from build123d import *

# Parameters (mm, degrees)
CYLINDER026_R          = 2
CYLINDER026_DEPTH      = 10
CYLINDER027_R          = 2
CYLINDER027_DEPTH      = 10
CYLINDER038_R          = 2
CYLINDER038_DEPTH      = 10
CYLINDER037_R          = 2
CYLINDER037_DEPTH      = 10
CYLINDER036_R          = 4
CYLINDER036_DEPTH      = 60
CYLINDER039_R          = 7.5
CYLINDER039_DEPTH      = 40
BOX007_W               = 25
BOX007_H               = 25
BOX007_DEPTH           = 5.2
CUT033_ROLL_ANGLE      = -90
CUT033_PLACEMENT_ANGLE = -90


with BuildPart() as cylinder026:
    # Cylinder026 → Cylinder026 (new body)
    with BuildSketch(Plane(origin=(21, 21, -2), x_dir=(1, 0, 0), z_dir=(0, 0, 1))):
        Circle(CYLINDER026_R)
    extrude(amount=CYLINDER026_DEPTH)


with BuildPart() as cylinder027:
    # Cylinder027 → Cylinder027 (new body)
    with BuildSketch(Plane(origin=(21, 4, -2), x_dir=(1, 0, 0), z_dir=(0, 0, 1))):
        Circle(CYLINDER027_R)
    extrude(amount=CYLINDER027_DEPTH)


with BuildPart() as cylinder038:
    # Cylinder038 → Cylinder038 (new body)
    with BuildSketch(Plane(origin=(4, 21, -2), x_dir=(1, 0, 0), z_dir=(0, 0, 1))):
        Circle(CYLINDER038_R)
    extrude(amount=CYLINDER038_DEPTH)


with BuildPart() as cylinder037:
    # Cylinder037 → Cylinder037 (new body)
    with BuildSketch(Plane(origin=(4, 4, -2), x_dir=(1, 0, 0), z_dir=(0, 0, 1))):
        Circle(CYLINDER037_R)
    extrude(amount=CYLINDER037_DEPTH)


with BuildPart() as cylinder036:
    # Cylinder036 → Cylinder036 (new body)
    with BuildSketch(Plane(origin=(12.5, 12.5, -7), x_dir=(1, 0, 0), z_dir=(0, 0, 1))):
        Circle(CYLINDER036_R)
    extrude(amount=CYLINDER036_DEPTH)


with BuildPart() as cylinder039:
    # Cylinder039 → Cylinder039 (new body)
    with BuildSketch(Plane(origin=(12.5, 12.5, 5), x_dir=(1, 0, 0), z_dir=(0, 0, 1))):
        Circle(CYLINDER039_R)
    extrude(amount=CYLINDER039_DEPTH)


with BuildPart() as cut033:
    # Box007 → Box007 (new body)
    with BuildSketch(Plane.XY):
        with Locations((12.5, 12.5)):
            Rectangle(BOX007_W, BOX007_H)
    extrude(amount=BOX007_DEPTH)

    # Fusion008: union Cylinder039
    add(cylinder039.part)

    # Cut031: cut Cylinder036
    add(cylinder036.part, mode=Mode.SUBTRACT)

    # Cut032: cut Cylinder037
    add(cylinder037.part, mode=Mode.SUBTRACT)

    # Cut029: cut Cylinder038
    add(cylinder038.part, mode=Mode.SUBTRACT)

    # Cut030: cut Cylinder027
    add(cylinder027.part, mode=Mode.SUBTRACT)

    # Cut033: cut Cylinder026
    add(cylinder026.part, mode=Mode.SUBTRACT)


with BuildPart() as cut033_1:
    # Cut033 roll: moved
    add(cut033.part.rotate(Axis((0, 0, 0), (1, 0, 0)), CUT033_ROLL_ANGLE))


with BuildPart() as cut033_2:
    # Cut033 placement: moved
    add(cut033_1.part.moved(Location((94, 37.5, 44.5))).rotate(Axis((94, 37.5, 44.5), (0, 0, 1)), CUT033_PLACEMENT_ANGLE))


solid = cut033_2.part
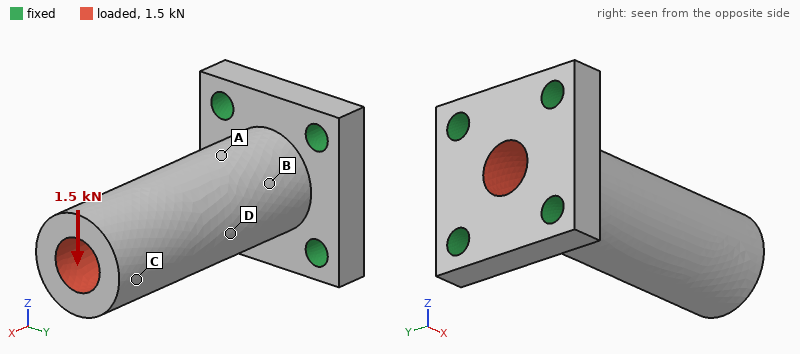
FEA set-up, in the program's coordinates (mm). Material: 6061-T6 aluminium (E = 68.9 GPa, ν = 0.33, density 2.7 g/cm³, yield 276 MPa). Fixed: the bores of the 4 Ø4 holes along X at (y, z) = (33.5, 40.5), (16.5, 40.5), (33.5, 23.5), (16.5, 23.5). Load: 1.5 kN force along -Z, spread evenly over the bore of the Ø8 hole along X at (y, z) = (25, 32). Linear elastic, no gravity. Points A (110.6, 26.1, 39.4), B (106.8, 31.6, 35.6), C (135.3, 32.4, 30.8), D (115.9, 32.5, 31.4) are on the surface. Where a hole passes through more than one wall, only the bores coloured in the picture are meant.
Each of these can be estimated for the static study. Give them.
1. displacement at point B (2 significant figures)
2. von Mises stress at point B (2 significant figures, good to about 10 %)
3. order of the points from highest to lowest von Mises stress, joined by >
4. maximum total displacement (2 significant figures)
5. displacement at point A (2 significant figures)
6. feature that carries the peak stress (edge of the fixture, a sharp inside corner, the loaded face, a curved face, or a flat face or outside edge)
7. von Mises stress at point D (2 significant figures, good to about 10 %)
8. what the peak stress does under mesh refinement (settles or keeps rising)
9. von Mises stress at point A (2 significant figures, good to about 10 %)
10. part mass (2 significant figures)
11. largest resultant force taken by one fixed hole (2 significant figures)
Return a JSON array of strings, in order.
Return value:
["0.019 mm", "31 MPa", "A > B > D > C", "0.13 mm", "0.035 mm", "edge of the fixture", "17 MPa", "keeps rising", "43 MPa", "21 g", "1.1 kN"]
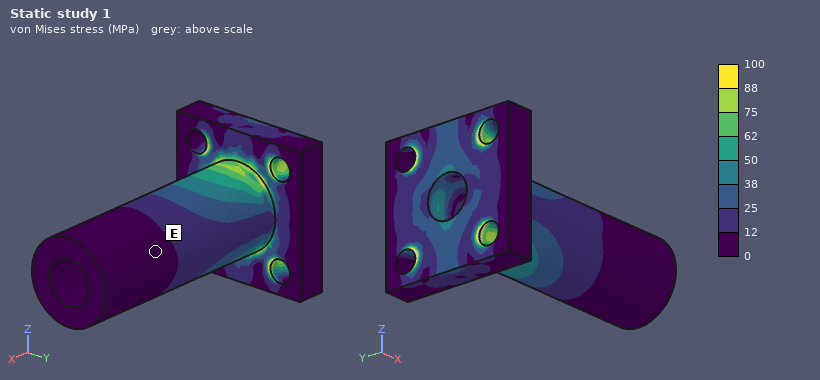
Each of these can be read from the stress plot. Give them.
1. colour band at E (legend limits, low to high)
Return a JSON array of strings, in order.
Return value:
["0 to 12 MPa"]
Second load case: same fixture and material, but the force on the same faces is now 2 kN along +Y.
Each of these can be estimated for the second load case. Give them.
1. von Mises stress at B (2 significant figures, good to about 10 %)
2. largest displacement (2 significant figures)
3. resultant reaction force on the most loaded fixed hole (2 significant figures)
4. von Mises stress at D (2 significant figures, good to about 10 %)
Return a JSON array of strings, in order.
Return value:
["64 MPa", "0.17 mm", "1.5 kN", "38 MPa"]
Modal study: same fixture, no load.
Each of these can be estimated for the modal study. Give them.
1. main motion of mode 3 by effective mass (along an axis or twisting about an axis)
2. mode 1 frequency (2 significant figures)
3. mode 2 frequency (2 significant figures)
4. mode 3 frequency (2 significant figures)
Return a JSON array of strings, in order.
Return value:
["twisting about X", "5400 Hz", "5400 Hz", "18 kHz"]
